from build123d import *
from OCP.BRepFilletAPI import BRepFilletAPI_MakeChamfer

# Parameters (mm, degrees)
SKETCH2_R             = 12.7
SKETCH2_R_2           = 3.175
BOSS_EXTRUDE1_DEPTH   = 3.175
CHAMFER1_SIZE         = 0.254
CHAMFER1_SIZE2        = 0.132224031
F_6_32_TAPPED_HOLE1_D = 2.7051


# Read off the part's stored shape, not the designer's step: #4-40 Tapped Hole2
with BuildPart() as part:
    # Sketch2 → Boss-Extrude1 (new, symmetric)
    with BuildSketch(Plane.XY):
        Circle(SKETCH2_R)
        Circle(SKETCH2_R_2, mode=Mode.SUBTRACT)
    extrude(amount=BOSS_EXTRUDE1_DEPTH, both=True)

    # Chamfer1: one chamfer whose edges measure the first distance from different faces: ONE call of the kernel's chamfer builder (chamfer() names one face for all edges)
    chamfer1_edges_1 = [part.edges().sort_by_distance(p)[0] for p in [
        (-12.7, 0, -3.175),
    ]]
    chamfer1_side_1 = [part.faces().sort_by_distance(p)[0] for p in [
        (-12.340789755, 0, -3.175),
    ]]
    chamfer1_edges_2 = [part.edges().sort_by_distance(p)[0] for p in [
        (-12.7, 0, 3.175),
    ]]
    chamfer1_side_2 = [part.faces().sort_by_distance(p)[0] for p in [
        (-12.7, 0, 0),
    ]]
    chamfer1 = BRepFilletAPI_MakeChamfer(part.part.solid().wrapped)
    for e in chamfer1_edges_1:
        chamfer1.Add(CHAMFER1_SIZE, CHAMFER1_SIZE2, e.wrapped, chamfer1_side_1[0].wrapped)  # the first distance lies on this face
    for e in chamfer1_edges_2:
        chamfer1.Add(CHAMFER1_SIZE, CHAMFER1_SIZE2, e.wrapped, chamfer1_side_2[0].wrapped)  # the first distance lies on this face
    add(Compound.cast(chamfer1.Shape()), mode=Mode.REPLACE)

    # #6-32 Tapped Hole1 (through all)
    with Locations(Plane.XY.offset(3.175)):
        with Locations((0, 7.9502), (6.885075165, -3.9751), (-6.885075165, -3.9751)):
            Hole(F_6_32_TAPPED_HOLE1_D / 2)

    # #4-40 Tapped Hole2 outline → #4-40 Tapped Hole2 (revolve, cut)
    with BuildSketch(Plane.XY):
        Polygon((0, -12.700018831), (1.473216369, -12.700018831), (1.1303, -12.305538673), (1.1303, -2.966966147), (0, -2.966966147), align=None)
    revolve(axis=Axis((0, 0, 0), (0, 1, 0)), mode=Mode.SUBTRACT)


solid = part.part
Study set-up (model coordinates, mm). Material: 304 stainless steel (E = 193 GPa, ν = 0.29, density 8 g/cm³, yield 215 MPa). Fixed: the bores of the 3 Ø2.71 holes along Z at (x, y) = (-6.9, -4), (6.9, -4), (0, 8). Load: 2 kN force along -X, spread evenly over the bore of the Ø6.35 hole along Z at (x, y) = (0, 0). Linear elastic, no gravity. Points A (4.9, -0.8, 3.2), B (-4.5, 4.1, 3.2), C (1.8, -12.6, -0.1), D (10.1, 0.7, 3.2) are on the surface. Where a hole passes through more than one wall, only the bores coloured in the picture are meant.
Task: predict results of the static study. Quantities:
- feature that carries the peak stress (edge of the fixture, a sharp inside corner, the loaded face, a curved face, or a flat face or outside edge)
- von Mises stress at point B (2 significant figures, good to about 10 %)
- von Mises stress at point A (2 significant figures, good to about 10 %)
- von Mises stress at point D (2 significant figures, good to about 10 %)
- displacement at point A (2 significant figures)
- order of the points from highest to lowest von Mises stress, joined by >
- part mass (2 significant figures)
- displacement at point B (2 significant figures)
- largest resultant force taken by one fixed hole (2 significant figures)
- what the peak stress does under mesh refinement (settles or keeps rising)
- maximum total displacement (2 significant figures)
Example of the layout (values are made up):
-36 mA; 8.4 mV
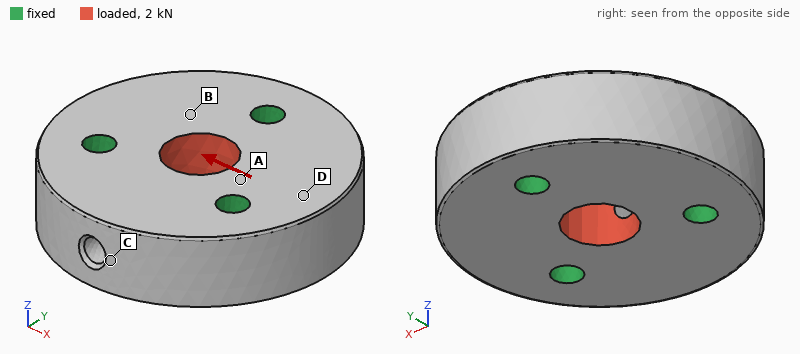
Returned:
edge of the fixture; 11 MPa; 16 MPa; 6.6 MPa; 0.42 µm; A > B > D > C; 23 g; 0.48 µm; 700 N; keeps rising; 0.73 µm
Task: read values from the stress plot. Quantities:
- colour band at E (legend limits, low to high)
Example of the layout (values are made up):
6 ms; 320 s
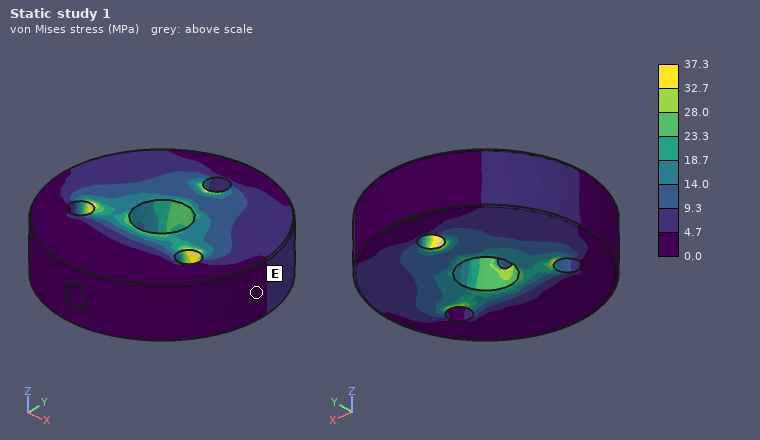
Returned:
0.0 to 4.7 MPa
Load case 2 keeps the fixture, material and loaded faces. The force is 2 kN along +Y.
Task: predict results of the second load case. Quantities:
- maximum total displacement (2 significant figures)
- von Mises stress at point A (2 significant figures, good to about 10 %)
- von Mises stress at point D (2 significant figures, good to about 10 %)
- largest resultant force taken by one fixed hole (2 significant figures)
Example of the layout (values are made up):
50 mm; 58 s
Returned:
0.78 µm; 13 MPa; 3.6 MPa; 680 N
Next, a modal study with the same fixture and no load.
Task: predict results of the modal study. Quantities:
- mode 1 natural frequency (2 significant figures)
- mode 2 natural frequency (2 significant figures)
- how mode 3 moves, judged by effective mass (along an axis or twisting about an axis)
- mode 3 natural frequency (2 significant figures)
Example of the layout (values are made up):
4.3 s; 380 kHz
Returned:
51 kHz; 52 kHz; along Z; 58 kHz
